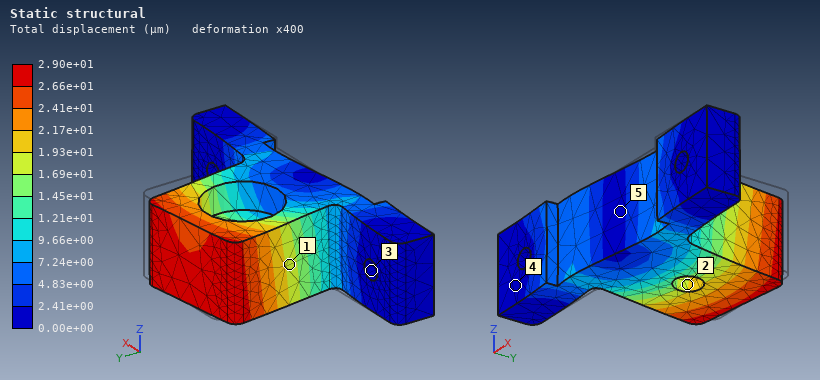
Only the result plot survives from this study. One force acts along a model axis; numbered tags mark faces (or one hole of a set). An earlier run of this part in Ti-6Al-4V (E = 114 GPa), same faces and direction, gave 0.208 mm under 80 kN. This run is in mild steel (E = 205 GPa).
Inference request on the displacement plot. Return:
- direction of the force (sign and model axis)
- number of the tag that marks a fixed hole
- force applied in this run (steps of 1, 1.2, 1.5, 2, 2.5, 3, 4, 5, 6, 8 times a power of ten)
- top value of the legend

-X
3
20 kN
2.90e+01 µm
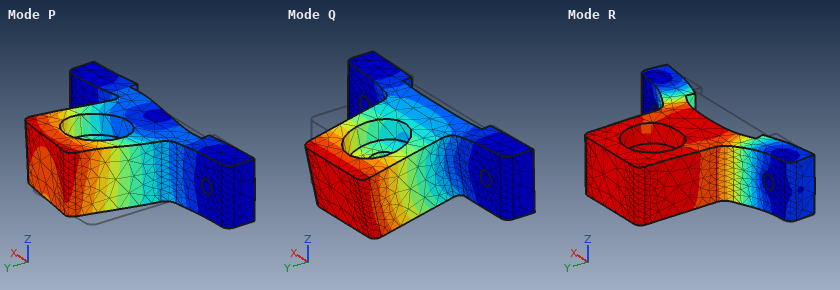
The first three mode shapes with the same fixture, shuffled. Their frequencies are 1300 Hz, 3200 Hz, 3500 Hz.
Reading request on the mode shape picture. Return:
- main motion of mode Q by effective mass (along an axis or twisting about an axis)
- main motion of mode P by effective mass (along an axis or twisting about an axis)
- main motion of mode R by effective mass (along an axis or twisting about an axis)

along Z
along X
along Y
